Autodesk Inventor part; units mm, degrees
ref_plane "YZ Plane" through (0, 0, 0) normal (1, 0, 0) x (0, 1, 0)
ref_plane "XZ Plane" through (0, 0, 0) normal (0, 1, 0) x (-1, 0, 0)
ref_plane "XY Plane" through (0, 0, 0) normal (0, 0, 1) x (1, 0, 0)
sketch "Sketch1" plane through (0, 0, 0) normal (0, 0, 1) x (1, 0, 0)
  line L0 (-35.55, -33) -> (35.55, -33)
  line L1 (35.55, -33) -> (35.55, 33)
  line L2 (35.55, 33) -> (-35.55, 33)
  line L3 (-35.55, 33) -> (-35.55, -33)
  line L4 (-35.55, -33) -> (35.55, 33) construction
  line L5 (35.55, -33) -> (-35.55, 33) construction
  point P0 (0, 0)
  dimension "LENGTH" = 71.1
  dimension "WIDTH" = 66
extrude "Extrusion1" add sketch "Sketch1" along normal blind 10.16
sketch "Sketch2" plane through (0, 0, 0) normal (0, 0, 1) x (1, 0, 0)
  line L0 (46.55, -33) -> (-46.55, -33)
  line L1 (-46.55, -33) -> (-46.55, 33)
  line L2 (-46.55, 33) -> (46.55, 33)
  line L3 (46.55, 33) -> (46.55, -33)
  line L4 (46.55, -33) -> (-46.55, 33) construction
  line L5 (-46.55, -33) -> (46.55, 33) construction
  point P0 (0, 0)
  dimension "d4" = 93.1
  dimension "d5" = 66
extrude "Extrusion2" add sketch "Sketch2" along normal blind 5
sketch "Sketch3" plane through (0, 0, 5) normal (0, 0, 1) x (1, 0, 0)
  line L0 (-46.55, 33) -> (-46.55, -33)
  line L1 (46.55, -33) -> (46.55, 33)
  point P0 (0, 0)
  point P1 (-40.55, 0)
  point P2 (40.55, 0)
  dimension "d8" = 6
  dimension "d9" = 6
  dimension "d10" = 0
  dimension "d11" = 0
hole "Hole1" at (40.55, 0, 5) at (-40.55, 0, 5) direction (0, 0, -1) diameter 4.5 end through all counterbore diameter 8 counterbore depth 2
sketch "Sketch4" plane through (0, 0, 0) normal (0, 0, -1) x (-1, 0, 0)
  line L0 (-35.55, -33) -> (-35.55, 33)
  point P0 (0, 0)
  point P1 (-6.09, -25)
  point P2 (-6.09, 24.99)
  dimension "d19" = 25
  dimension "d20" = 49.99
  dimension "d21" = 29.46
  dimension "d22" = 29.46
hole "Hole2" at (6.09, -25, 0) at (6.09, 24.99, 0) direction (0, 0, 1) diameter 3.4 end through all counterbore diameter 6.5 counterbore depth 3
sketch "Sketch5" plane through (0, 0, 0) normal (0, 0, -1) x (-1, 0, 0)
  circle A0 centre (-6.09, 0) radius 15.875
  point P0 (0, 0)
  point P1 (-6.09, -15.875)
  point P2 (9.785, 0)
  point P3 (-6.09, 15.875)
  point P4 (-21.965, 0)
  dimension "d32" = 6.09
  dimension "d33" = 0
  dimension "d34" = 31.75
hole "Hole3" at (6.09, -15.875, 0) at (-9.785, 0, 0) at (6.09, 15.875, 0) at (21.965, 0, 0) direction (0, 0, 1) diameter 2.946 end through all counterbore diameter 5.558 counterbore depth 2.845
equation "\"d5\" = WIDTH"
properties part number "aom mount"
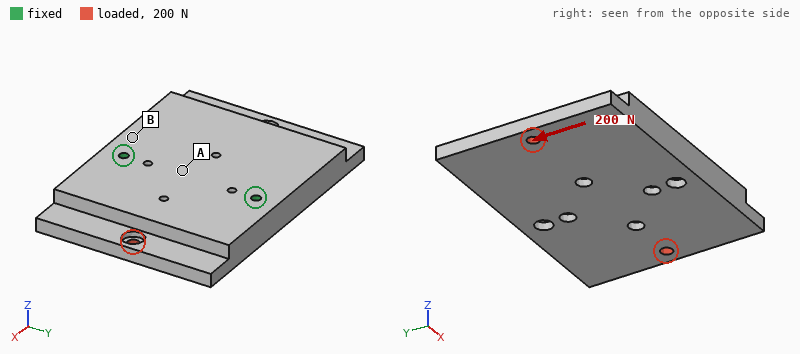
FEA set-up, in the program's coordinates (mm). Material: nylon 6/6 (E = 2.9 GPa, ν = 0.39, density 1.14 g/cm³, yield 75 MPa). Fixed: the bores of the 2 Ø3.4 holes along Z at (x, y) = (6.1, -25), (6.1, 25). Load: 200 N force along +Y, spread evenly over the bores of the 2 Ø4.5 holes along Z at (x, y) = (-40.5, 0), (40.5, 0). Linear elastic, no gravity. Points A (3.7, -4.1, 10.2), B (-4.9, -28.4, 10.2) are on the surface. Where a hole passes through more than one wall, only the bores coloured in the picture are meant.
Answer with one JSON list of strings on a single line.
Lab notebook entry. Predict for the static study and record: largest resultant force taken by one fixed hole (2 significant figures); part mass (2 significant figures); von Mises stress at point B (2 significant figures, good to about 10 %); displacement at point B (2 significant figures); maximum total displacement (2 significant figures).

["100 N", "61 g", "0.59 MPa", "5.3 µm", "23 µm"]
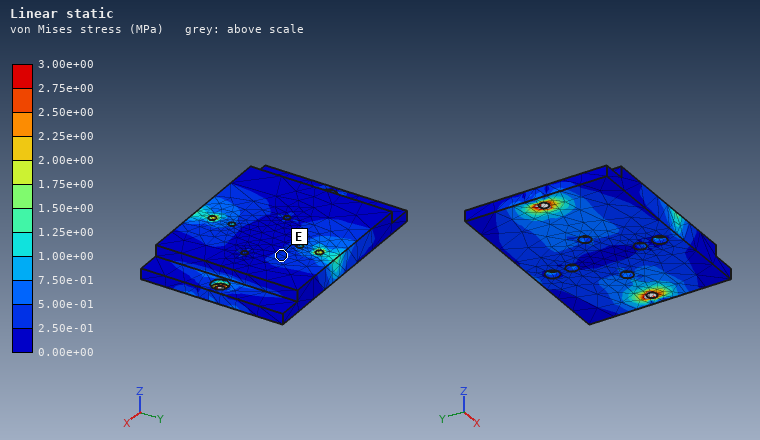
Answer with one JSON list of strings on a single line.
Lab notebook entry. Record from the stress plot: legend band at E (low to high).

["2.50e-01 to 5.00e-01 MPa"]
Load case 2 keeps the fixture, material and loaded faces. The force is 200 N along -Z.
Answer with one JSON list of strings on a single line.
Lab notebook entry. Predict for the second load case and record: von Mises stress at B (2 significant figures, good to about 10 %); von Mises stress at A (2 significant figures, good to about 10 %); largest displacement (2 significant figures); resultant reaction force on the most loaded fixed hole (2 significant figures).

["3.3 MPa", "3.3 MPa", "0.42 mm", "110 N"]
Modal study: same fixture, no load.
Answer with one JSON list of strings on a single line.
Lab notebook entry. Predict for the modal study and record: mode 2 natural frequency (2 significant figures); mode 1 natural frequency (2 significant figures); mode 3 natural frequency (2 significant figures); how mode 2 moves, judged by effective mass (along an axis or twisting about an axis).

["1400 Hz", "660 Hz", "1700 Hz", "along Z"]
